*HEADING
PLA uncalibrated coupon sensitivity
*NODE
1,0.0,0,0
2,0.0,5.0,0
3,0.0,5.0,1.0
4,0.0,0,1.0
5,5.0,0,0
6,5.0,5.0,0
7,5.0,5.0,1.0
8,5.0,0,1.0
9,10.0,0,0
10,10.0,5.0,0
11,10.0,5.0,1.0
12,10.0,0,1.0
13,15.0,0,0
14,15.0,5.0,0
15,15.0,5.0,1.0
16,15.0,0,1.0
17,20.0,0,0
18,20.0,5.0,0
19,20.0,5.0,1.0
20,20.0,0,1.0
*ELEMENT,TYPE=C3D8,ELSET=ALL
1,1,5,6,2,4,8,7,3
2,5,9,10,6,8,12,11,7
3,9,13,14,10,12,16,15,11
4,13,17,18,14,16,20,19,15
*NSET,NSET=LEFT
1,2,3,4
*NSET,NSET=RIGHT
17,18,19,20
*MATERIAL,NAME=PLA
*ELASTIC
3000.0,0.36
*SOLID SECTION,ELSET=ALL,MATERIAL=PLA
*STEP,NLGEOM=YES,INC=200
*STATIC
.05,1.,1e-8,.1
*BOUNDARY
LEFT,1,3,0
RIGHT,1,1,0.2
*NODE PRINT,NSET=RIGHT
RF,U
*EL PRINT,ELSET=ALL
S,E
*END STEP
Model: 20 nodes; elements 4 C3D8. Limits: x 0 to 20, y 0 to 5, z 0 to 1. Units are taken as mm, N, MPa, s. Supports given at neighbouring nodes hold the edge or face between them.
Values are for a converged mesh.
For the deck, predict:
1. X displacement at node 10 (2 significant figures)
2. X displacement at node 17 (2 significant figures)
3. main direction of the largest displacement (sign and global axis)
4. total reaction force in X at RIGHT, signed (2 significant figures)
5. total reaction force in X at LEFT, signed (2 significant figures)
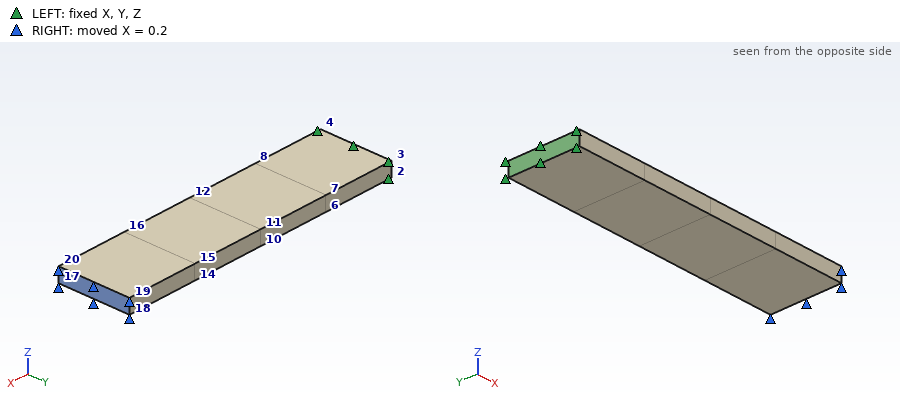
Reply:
0.098 mm
0.20 mm
+X
150 N
-150 N
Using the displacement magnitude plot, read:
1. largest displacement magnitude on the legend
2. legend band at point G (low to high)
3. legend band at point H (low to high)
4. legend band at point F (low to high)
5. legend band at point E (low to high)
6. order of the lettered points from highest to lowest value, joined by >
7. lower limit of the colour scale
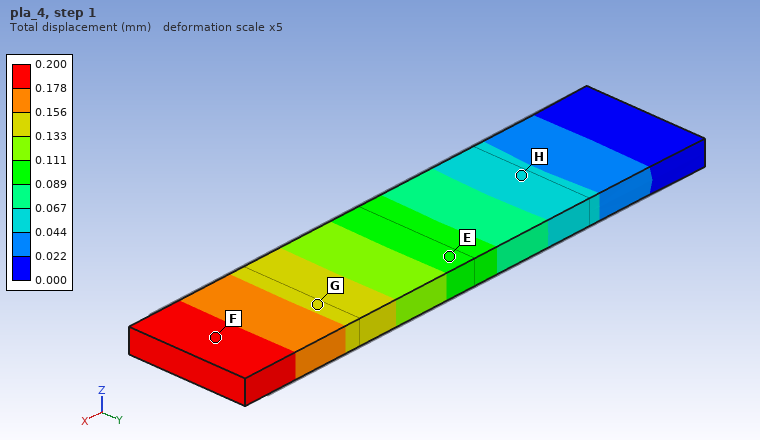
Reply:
0.200 mm
0.133 to 0.156 mm
0.044 to 0.067 mm
0.178 to 0.200 mm
0.089 to 0.111 mm
F > G > E > H
0.000 mm
